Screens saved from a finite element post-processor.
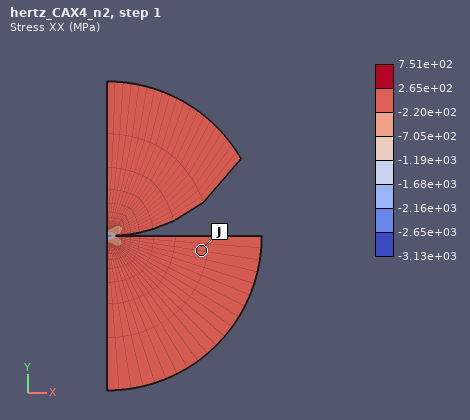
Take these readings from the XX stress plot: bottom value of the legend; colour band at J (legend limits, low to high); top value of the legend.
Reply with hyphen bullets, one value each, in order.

- -3.13e+03 MPa
- -2.20e+02 to 2.65e+02 MPa
- 7.51e+02 MPa
